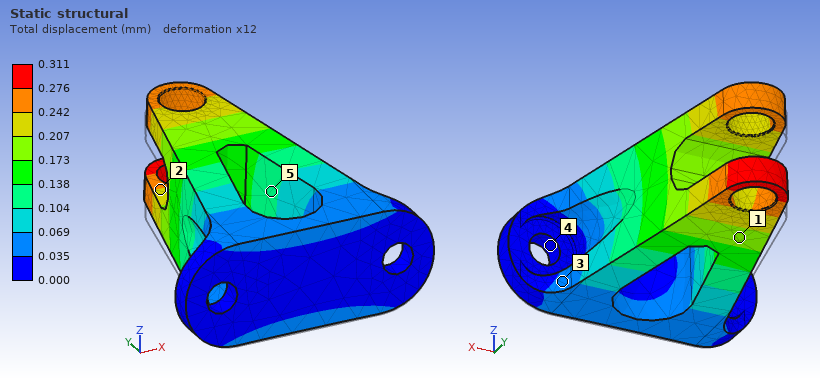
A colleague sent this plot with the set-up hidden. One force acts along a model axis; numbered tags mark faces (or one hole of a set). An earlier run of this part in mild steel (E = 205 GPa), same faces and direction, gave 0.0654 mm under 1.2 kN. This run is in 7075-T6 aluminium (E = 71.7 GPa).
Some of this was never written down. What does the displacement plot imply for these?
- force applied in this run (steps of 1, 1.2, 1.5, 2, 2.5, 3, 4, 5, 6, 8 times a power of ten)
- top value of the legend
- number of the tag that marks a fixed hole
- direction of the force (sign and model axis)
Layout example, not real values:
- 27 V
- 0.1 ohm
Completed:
- 2 kN
- 0.311 mm
- 4
- +Z
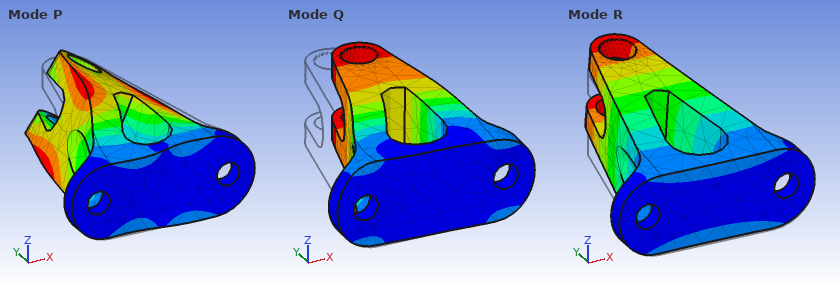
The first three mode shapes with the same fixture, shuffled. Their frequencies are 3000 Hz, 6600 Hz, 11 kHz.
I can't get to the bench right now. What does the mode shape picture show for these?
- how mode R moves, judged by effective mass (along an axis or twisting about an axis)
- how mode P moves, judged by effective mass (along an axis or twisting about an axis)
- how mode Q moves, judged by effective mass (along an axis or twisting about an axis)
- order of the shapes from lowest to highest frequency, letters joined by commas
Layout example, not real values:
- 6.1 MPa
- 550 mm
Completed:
- along Z
- twisting about Y
- along X
- R, Q, P
